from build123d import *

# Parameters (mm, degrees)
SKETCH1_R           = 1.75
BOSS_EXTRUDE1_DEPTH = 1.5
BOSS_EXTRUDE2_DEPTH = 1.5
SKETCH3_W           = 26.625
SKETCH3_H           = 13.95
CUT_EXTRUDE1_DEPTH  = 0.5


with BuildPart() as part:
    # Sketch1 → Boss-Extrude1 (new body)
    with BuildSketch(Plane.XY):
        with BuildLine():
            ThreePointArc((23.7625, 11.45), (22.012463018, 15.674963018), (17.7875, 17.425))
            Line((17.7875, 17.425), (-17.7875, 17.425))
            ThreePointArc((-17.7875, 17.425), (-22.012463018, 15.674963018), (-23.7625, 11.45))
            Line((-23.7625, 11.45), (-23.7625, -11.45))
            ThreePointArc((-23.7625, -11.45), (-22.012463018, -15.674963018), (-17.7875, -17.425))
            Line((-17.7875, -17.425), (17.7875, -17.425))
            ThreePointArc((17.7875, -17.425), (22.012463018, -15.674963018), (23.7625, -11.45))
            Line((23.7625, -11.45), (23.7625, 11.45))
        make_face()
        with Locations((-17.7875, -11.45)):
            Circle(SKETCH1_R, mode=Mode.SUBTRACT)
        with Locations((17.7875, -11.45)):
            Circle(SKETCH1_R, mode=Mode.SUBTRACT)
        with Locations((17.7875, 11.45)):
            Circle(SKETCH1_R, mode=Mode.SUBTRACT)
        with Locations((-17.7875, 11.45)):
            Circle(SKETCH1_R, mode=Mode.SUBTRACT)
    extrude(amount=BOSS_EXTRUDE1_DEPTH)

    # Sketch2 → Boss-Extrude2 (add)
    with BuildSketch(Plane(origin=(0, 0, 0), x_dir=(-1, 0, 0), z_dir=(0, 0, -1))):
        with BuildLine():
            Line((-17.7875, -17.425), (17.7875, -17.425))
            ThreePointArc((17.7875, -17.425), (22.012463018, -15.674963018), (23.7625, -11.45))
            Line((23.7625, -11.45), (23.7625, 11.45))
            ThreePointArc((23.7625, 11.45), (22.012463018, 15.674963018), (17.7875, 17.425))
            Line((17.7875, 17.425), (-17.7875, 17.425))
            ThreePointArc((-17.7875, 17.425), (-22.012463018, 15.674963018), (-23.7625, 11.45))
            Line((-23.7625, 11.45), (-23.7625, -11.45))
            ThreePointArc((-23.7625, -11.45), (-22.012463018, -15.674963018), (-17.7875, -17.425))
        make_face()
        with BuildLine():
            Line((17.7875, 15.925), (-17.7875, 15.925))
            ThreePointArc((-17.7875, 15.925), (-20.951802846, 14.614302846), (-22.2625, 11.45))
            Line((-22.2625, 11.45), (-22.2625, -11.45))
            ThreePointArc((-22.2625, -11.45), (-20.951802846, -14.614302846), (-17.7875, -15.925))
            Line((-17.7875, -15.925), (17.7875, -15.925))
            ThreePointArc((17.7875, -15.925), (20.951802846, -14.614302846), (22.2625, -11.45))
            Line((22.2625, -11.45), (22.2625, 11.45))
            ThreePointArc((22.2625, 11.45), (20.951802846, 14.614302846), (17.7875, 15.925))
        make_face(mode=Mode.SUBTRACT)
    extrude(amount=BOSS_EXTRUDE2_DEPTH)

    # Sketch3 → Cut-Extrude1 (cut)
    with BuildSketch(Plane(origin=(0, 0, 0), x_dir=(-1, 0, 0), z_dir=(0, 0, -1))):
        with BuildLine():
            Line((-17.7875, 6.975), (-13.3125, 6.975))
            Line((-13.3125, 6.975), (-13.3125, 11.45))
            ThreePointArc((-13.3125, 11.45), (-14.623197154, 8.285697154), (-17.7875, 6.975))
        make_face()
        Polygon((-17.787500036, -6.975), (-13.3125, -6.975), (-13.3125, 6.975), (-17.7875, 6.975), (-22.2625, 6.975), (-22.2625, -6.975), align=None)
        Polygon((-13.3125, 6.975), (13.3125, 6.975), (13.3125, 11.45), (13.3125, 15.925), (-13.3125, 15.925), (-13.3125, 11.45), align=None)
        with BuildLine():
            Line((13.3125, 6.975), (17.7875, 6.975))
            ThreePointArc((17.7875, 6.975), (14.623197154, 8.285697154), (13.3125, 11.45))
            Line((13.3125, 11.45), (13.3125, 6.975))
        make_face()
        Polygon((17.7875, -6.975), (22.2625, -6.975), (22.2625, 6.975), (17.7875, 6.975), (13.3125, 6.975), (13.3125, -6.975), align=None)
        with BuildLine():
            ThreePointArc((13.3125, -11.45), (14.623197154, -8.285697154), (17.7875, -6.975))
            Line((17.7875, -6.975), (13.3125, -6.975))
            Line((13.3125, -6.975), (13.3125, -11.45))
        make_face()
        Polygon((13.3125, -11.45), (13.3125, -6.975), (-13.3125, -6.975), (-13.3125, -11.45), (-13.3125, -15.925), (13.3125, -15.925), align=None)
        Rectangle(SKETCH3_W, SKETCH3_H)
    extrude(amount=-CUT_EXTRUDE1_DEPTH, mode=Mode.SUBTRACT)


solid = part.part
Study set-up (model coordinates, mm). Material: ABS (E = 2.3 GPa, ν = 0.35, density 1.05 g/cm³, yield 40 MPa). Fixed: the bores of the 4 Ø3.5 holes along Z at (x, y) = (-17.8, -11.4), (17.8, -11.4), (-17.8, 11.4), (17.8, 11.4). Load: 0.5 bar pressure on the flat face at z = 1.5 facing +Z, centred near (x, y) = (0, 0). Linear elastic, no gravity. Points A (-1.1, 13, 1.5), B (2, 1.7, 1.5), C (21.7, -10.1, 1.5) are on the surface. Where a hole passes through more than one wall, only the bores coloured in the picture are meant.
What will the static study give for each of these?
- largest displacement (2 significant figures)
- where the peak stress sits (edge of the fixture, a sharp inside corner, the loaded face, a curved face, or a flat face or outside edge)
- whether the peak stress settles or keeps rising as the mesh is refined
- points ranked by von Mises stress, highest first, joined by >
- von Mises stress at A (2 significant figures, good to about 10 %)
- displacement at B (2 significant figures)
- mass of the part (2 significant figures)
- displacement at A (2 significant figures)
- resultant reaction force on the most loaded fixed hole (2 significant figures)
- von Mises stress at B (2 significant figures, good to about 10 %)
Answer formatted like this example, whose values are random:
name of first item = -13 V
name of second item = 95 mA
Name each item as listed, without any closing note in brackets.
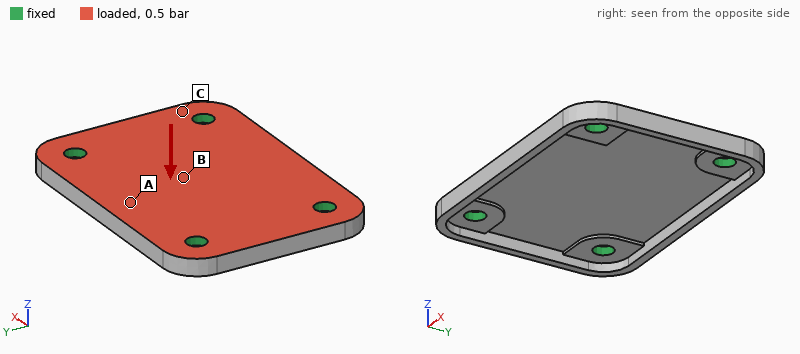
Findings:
largest displacement = 0.59 mm
where the peak stress sits = edge of the fixture
whether the peak stress settles or keeps rising as the mesh is refined = keeps rising
points ranked by von Mises stress, highest first, joined by > = B > A > C
von Mises stress at A = 5.6 MPa
displacement at B = 0.57 mm
mass of the part = 2.3 g
displacement at A = 0.29 mm
resultant reaction force on the most loaded fixed hole = 23 N
von Mises stress at B = 9.7 MPa
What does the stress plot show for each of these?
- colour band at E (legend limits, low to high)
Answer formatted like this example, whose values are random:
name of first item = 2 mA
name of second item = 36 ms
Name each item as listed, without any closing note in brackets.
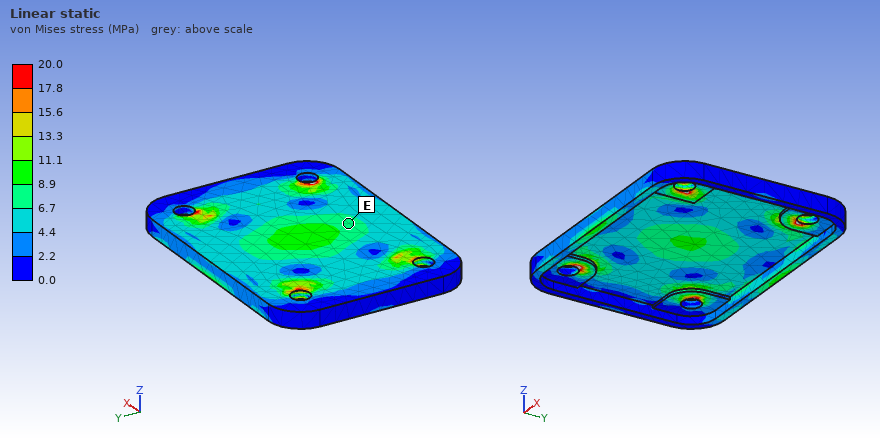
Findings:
colour band at E = 6.7 to 8.9 MPa
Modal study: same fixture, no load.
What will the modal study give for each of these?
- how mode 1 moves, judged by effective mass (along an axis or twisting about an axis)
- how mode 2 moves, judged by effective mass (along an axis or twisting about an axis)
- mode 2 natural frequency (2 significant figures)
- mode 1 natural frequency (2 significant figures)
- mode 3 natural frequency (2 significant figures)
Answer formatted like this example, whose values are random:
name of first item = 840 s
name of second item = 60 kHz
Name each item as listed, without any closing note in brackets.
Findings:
how mode 1 moves, judged by effective mass = along Z
how mode 2 moves, judged by effective mass = twisting about X
mode 2 natural frequency = 2600 Hz
mode 1 natural frequency = 1800 Hz
mode 3 natural frequency = 3100 Hz
